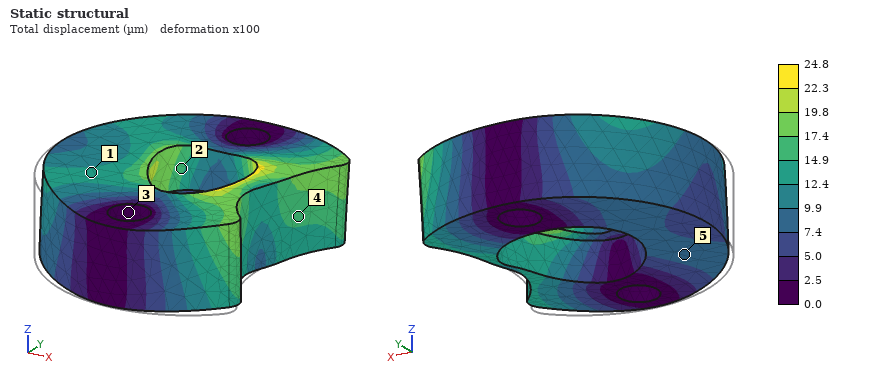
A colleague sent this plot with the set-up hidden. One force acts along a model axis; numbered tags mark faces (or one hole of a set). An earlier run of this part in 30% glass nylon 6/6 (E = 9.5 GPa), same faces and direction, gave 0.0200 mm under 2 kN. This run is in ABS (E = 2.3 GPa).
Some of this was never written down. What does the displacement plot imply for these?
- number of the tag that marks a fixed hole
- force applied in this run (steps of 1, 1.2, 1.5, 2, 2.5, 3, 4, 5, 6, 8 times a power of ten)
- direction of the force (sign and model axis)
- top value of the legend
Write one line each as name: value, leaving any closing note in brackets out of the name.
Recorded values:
number of the tag that marks a fixed hole: 3
force applied in this run: 600 N
direction of the force: +Y
top value of the legend: 24.8 µm
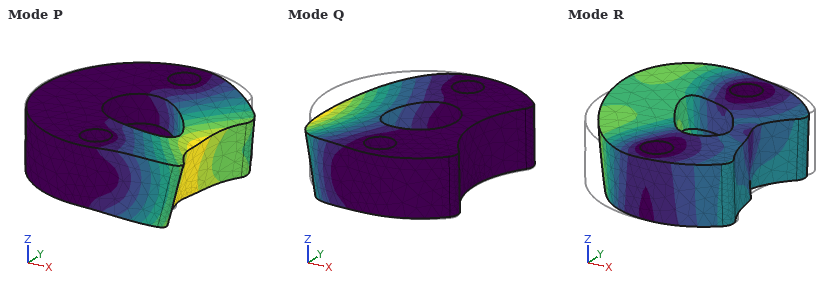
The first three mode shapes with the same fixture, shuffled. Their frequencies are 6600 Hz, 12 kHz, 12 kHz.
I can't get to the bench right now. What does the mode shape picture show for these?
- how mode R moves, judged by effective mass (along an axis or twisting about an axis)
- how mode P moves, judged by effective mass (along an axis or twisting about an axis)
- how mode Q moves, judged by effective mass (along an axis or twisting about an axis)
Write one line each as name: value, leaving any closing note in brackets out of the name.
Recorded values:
how mode R moves, judged by effective mass: along Y
how mode P moves, judged by effective mass: along Z
how mode Q moves, judged by effective mass: along Z
